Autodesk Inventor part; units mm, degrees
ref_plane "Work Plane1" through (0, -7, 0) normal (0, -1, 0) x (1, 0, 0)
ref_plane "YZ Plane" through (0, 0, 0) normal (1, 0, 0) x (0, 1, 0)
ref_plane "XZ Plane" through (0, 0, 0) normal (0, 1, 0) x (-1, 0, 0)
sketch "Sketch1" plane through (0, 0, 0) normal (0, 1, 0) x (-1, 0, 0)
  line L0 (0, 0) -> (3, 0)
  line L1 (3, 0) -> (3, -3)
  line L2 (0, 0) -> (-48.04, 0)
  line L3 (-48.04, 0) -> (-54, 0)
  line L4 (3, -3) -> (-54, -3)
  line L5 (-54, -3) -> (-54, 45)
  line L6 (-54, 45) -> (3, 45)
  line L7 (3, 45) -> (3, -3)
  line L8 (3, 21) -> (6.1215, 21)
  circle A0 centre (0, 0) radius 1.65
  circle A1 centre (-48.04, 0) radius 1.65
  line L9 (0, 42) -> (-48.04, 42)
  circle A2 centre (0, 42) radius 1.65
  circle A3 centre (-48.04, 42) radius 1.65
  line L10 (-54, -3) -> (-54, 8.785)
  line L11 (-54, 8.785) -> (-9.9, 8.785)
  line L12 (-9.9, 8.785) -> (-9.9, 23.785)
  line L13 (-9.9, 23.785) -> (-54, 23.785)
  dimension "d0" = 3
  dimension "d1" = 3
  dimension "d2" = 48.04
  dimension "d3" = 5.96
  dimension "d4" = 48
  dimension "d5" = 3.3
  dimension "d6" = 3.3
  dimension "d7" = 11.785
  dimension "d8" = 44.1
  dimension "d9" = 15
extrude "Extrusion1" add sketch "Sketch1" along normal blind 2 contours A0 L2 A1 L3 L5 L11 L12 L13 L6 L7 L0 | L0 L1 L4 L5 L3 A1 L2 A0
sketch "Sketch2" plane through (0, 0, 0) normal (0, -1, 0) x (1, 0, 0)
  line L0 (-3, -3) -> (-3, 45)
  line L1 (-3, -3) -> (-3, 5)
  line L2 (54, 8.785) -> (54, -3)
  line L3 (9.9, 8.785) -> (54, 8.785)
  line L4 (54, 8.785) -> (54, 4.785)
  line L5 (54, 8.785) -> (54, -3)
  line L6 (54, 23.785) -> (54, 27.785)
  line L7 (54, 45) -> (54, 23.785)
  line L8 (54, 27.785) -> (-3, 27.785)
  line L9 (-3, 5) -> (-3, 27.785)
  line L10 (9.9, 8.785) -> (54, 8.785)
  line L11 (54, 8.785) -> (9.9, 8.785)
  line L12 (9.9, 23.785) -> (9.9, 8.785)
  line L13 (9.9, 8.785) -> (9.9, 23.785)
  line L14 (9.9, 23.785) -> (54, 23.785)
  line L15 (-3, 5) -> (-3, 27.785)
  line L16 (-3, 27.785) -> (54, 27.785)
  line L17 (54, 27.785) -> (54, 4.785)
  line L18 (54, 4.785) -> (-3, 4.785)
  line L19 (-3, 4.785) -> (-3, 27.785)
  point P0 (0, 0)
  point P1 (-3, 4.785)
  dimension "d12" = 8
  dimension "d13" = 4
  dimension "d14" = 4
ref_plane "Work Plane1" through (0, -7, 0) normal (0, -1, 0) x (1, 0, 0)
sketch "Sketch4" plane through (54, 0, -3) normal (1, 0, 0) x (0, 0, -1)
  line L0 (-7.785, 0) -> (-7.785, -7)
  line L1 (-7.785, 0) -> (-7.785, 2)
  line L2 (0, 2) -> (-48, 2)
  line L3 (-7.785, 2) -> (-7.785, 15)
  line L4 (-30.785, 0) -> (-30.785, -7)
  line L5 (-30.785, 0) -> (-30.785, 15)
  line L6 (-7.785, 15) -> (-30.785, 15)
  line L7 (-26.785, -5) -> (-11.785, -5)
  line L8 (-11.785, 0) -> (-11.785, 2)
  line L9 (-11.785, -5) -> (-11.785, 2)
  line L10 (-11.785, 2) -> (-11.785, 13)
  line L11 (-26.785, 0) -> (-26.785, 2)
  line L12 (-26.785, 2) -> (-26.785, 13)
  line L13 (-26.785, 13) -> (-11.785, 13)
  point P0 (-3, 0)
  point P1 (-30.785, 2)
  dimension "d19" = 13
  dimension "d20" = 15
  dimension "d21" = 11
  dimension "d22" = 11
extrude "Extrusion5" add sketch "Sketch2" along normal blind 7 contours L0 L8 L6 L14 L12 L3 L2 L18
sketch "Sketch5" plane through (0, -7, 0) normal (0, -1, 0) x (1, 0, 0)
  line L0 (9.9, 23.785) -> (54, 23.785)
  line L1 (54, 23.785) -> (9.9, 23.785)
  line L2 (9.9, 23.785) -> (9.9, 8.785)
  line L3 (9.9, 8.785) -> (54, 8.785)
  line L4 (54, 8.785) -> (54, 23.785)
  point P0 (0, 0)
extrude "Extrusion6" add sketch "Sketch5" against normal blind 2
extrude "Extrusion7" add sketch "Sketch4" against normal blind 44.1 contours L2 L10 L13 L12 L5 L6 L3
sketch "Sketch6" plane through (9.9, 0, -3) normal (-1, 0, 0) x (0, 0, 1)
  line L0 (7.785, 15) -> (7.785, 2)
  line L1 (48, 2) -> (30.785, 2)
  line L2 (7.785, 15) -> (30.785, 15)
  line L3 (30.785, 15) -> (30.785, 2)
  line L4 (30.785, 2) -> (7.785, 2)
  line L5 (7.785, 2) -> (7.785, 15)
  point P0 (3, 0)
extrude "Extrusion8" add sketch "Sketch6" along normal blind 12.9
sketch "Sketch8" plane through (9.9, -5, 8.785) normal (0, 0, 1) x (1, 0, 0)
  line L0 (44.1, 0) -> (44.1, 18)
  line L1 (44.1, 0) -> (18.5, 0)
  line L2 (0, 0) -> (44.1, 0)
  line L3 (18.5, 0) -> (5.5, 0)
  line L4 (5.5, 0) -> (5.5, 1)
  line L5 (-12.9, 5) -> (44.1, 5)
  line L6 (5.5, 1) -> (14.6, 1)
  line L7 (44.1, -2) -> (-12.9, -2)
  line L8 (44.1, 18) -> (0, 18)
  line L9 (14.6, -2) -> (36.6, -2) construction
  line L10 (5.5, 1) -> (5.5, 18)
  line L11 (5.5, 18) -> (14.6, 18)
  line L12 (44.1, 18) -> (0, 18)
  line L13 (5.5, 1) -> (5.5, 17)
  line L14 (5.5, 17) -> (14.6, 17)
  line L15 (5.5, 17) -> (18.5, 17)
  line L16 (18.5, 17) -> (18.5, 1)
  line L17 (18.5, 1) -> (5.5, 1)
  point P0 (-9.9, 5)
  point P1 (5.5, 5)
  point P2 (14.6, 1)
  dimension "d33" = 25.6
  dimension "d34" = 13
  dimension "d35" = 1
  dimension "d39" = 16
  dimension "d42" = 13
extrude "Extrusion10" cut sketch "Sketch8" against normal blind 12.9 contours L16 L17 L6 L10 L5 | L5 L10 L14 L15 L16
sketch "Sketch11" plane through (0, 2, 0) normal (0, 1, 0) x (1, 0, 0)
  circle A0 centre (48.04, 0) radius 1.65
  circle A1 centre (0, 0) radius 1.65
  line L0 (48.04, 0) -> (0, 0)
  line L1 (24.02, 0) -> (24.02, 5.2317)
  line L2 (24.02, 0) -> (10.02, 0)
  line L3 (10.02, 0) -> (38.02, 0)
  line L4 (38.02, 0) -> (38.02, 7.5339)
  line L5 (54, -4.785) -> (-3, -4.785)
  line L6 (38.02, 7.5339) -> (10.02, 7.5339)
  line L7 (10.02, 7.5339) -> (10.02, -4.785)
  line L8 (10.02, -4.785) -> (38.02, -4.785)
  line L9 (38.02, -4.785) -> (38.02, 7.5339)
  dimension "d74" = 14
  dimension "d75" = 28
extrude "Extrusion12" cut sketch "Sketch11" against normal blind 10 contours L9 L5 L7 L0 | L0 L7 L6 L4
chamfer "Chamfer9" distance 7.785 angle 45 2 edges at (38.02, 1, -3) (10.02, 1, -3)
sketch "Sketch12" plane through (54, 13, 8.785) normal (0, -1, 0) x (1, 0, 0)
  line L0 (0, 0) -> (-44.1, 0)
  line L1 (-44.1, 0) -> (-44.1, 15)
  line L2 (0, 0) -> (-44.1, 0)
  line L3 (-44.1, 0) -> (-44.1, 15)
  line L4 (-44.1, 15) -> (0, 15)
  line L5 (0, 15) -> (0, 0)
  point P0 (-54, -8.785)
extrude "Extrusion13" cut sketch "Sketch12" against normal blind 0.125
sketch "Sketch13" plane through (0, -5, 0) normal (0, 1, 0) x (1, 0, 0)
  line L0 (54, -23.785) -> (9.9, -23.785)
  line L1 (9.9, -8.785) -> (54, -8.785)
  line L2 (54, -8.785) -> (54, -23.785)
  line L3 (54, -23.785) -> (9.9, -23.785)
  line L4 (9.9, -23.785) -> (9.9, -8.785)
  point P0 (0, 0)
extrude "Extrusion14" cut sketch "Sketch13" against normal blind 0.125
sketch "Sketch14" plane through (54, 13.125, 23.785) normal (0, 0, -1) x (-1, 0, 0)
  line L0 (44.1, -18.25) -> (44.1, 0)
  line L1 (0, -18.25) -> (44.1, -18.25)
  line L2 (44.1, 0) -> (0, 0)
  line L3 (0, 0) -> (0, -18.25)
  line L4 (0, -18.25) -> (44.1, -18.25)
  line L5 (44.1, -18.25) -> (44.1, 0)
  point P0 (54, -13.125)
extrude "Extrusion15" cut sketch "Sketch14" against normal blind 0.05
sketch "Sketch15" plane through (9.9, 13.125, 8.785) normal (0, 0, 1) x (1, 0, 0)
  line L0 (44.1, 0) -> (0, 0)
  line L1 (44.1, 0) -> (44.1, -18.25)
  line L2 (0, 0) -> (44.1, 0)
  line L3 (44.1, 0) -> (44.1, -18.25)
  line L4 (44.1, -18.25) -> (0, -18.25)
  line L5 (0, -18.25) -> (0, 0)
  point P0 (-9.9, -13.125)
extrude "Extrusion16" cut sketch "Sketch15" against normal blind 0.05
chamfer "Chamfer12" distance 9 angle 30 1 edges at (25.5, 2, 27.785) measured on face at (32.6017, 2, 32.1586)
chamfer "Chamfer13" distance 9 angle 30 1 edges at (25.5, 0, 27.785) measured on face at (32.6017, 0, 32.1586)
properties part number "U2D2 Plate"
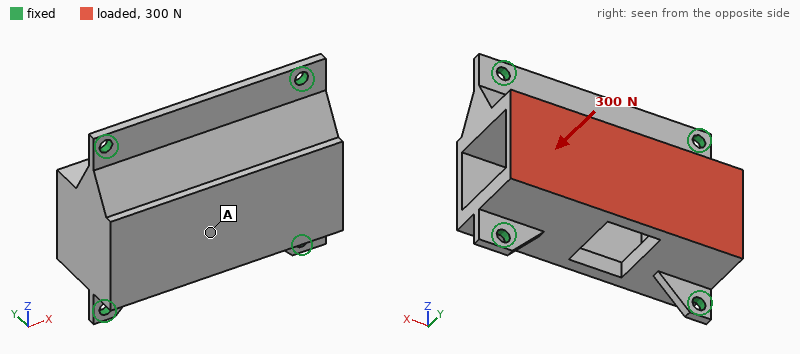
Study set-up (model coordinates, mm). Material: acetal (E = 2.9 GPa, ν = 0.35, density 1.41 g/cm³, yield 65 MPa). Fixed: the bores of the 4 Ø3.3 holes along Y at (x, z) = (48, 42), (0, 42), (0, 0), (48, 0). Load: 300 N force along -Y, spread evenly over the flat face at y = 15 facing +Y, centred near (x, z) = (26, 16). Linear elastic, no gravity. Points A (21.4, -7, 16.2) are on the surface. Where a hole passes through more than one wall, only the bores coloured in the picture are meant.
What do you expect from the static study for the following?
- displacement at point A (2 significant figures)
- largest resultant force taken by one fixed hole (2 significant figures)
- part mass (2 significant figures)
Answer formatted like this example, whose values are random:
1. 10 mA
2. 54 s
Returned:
1. 0.079 mm
2. 97 N
3. 29 g
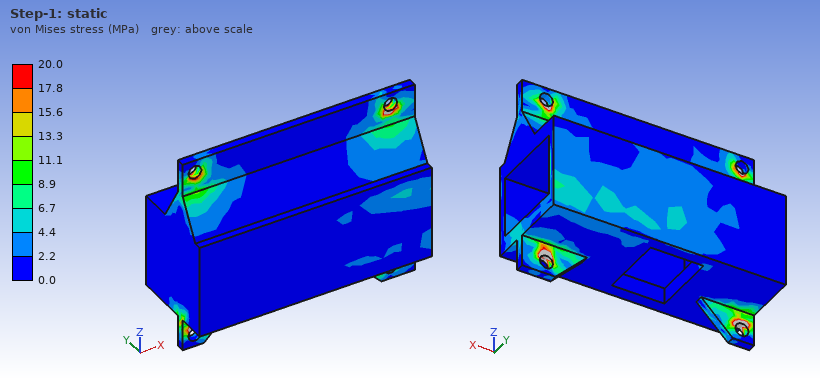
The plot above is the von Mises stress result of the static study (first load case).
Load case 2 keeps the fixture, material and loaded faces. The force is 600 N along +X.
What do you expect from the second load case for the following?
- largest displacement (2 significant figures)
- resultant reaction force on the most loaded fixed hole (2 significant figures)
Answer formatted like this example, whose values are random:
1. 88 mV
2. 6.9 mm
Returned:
1. 0.22 mm
2. 210 N
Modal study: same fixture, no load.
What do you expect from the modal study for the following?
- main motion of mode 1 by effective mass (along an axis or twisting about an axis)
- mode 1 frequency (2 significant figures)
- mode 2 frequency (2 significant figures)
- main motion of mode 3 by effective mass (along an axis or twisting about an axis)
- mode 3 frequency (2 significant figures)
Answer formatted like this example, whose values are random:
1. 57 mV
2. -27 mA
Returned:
1. along Y
2. 1800 Hz
3. 2300 Hz
4. along Z
5. 2900 Hz
